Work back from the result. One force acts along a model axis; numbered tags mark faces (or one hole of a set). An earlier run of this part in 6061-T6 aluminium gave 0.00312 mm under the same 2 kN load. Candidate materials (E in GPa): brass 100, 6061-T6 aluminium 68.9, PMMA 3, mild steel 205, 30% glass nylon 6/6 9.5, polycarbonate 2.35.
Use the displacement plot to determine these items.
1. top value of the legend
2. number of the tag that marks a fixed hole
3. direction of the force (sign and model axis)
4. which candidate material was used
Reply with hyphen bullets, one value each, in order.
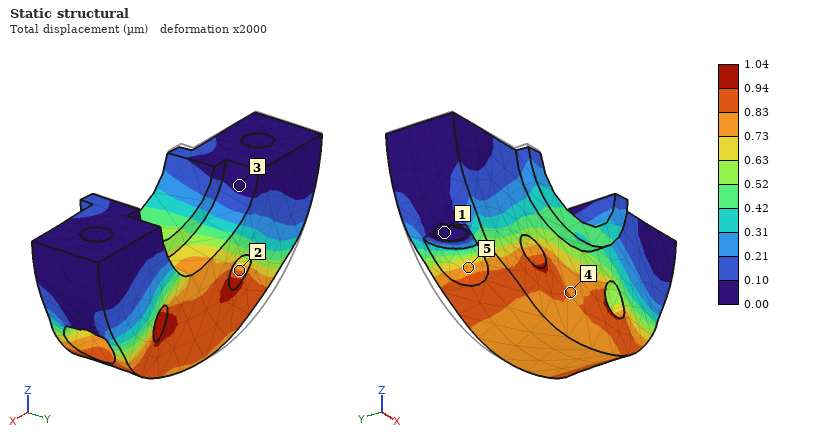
- 1.04 µm
- 1
- +X
- mild steel
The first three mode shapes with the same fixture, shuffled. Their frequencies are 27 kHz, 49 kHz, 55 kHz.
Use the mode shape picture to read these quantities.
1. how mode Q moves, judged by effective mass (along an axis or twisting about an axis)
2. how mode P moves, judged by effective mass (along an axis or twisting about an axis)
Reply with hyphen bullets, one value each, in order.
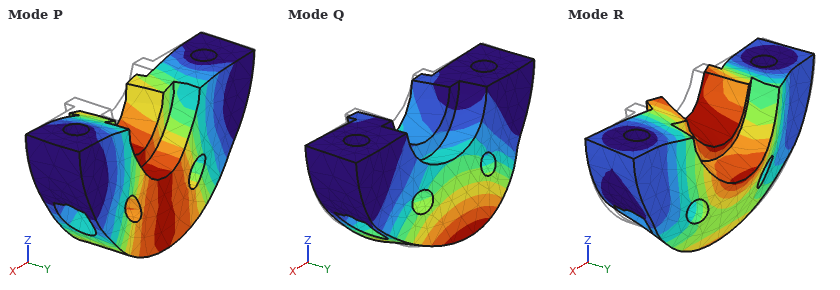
- along Y
- along Z
